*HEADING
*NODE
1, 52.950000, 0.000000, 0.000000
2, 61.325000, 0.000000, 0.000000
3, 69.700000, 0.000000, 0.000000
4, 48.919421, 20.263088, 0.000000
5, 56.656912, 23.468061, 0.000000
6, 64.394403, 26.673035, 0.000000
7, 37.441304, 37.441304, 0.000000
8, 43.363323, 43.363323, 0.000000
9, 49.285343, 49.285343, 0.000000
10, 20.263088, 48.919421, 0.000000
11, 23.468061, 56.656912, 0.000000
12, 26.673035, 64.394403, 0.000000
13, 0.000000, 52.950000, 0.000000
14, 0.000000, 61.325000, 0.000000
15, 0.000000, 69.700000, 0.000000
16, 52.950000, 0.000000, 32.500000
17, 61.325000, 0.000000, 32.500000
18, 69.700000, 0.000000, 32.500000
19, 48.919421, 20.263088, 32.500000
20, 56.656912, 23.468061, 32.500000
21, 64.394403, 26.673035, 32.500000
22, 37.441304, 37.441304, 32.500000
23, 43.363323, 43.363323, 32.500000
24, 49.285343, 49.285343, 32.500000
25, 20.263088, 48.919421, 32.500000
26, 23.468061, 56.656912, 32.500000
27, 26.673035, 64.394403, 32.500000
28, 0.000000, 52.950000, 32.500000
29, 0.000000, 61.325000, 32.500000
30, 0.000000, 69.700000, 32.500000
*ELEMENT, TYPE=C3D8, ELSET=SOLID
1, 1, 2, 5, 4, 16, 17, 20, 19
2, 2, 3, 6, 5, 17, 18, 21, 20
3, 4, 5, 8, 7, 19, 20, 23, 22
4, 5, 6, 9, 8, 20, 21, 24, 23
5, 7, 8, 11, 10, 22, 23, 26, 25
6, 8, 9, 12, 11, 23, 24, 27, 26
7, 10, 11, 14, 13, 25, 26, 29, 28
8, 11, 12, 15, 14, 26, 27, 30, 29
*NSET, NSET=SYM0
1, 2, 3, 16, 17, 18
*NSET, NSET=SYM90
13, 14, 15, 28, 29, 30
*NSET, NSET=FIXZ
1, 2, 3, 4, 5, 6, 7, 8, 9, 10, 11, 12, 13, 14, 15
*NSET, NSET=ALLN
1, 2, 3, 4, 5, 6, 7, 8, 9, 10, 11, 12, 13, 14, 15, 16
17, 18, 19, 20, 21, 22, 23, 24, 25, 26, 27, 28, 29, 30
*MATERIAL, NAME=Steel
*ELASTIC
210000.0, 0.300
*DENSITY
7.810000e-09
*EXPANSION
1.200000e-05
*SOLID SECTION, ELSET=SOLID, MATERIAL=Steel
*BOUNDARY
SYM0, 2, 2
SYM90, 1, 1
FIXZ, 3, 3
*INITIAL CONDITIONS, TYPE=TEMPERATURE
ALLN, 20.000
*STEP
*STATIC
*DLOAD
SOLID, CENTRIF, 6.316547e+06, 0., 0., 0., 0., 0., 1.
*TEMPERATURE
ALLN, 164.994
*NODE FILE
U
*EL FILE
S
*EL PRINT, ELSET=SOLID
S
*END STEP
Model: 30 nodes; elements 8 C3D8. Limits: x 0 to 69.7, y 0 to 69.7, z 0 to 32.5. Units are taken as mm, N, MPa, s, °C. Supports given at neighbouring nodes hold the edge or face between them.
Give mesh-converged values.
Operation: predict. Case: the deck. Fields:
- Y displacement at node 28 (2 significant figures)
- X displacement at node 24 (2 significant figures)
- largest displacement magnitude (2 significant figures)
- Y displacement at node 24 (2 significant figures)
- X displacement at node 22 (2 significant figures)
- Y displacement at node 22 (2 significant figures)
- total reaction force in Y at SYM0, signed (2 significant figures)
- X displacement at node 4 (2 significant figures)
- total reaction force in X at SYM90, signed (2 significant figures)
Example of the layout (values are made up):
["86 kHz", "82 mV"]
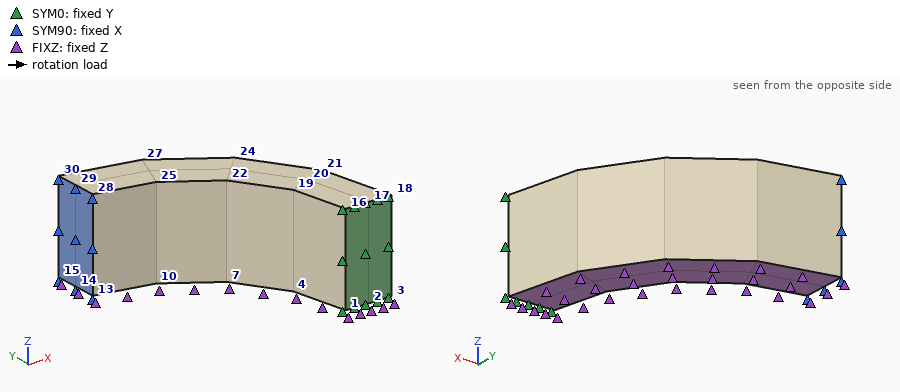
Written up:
["0.14 mm", "0.12 mm", "0.18 mm", "0.12 mm", "0.10 mm", "0.10 mm", "-98000 N", "0.14 mm", "-98000 N"]
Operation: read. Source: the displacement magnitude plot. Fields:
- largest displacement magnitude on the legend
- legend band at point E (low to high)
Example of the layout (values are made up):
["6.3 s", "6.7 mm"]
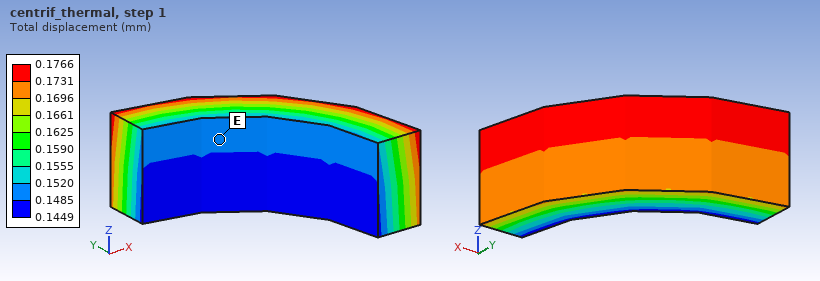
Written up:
["0.1766 mm", "0.1485 to 0.1520 mm"]
